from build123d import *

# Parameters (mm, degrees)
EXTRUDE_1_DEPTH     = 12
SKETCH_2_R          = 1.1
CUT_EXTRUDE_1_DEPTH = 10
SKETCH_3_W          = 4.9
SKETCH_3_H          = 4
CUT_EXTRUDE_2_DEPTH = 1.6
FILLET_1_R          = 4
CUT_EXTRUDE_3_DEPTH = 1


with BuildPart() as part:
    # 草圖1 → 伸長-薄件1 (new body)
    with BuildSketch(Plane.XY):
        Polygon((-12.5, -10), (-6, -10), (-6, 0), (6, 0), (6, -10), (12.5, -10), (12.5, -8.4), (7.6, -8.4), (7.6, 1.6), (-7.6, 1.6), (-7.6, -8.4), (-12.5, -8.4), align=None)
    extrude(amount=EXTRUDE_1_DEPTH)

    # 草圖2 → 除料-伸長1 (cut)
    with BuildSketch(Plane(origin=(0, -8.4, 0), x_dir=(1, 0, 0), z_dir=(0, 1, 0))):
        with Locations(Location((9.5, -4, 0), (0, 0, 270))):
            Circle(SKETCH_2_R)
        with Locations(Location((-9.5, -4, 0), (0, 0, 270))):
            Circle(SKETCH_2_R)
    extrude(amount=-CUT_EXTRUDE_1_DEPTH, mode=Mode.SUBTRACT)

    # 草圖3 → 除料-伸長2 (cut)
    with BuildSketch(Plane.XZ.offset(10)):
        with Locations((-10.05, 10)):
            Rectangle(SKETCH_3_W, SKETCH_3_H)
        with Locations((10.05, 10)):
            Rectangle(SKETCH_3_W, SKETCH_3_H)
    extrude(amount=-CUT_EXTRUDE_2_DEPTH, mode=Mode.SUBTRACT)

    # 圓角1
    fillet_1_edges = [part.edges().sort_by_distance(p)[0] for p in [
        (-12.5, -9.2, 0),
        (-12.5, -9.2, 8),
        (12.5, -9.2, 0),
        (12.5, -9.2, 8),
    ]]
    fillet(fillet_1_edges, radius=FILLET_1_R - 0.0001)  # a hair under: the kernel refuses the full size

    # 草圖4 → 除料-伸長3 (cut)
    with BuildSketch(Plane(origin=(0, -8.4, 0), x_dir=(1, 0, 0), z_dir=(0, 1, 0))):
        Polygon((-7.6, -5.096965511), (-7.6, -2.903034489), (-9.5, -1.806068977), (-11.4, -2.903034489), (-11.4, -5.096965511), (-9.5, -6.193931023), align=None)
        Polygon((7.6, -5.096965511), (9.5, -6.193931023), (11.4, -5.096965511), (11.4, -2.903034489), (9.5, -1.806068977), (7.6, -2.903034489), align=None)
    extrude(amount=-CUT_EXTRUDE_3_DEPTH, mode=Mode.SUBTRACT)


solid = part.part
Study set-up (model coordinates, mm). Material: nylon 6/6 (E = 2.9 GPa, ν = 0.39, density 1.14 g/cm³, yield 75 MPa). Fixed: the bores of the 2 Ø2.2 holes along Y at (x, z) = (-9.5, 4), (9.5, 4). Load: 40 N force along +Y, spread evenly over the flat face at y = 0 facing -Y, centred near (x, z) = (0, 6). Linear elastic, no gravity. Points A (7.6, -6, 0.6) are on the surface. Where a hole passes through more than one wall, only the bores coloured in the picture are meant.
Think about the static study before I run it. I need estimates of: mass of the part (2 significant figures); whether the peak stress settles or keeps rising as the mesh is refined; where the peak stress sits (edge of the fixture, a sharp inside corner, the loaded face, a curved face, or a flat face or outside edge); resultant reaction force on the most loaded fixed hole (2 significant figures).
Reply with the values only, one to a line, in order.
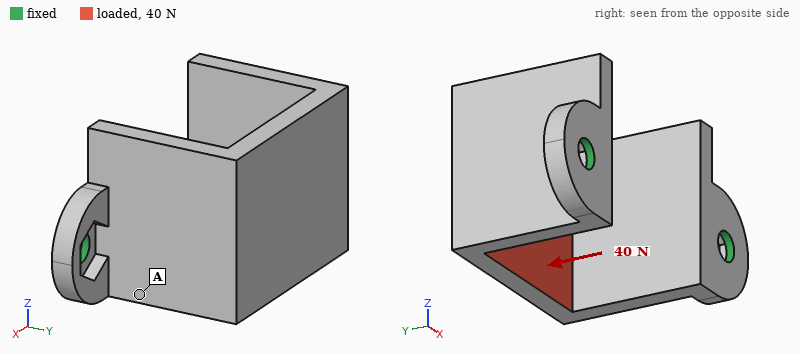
0.85 g
keeps rising
edge of the fixture
21 N
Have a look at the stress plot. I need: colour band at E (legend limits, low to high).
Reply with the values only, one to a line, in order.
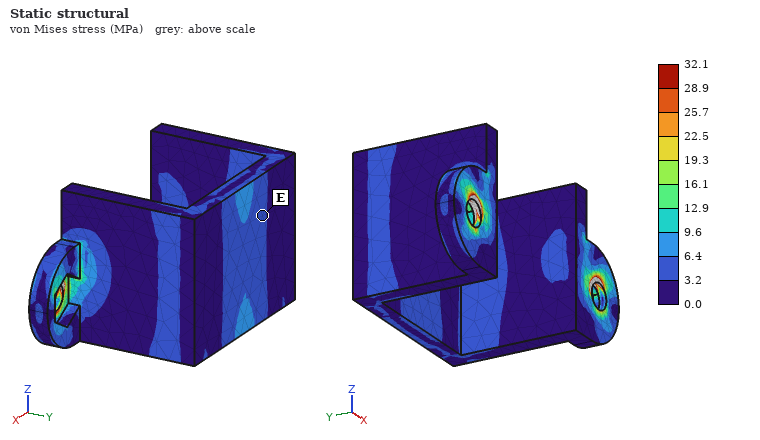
3.2 to 6.4 MPa
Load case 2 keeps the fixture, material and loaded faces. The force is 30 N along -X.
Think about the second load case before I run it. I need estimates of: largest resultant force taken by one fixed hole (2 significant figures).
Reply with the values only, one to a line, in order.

20 N
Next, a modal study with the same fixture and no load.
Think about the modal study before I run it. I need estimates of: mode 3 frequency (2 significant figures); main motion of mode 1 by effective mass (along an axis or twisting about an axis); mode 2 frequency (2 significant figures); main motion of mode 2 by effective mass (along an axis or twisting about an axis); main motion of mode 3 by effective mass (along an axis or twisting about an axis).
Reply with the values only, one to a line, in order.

3100 Hz
along Z
2300 Hz
along X
twisting about Y
